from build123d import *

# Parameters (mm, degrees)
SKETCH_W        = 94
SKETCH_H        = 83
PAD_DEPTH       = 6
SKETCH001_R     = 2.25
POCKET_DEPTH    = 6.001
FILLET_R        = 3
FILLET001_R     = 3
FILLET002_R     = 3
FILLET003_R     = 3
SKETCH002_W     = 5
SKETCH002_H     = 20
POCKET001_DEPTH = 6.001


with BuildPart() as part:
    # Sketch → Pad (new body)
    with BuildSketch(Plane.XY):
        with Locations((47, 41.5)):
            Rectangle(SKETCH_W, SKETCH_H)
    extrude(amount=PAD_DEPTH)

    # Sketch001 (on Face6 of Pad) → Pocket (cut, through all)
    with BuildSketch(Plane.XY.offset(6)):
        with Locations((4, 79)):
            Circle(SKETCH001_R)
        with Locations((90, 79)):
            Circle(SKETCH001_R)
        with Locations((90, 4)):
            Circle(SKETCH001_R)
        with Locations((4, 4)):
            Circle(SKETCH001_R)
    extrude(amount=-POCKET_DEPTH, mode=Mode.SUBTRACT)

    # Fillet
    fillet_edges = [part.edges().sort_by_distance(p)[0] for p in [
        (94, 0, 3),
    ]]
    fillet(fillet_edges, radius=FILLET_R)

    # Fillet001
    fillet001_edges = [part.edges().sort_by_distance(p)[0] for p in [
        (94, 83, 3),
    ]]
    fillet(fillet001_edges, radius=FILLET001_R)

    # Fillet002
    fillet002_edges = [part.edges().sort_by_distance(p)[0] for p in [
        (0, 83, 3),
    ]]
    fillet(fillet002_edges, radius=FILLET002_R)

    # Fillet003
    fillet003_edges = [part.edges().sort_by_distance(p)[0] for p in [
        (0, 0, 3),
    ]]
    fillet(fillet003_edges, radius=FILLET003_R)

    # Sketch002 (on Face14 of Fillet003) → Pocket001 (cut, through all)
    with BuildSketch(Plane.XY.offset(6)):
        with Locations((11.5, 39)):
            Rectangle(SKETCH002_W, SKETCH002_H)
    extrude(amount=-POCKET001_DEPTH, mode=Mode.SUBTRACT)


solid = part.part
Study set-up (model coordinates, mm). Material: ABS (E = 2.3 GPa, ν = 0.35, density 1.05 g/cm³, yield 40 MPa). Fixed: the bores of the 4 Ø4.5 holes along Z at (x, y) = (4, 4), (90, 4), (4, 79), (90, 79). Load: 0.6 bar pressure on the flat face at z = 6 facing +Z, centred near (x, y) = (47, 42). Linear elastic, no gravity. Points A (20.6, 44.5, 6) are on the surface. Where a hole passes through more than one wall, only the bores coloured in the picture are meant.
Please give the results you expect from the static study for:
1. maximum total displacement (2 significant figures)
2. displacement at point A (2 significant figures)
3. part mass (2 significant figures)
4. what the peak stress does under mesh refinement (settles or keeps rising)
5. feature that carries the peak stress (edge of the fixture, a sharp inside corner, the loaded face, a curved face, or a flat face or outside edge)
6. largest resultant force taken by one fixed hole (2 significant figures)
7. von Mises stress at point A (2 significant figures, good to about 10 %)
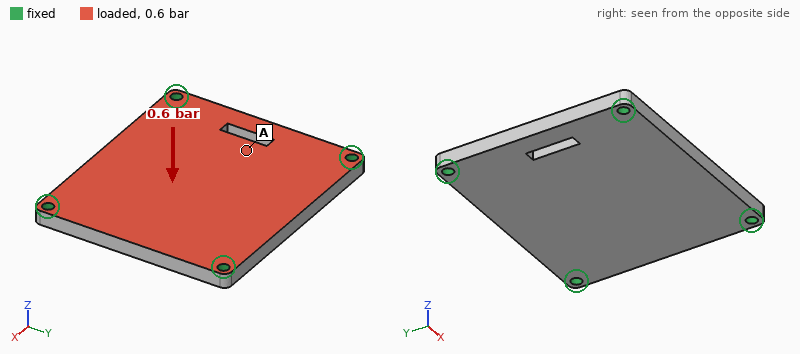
0.50 mm
0.37 mm
48 g
keeps rising
edge of the fixture
120 N
3.5 MPa
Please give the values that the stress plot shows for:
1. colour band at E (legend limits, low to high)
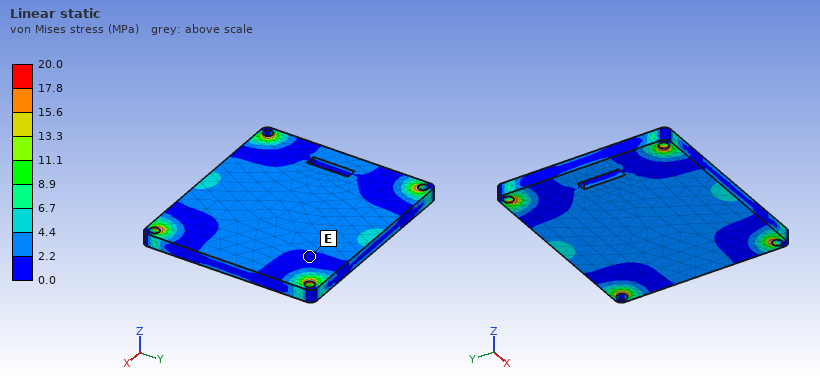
0.0 to 2.2 MPa
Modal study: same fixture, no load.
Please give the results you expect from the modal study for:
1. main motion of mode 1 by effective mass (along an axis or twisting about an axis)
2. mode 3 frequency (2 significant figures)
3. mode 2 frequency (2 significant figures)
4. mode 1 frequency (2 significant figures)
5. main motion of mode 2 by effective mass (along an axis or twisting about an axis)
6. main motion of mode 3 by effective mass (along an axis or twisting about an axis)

along Z
1600 Hz
1400 Hz
820 Hz
twisting about X
twisting about Y
